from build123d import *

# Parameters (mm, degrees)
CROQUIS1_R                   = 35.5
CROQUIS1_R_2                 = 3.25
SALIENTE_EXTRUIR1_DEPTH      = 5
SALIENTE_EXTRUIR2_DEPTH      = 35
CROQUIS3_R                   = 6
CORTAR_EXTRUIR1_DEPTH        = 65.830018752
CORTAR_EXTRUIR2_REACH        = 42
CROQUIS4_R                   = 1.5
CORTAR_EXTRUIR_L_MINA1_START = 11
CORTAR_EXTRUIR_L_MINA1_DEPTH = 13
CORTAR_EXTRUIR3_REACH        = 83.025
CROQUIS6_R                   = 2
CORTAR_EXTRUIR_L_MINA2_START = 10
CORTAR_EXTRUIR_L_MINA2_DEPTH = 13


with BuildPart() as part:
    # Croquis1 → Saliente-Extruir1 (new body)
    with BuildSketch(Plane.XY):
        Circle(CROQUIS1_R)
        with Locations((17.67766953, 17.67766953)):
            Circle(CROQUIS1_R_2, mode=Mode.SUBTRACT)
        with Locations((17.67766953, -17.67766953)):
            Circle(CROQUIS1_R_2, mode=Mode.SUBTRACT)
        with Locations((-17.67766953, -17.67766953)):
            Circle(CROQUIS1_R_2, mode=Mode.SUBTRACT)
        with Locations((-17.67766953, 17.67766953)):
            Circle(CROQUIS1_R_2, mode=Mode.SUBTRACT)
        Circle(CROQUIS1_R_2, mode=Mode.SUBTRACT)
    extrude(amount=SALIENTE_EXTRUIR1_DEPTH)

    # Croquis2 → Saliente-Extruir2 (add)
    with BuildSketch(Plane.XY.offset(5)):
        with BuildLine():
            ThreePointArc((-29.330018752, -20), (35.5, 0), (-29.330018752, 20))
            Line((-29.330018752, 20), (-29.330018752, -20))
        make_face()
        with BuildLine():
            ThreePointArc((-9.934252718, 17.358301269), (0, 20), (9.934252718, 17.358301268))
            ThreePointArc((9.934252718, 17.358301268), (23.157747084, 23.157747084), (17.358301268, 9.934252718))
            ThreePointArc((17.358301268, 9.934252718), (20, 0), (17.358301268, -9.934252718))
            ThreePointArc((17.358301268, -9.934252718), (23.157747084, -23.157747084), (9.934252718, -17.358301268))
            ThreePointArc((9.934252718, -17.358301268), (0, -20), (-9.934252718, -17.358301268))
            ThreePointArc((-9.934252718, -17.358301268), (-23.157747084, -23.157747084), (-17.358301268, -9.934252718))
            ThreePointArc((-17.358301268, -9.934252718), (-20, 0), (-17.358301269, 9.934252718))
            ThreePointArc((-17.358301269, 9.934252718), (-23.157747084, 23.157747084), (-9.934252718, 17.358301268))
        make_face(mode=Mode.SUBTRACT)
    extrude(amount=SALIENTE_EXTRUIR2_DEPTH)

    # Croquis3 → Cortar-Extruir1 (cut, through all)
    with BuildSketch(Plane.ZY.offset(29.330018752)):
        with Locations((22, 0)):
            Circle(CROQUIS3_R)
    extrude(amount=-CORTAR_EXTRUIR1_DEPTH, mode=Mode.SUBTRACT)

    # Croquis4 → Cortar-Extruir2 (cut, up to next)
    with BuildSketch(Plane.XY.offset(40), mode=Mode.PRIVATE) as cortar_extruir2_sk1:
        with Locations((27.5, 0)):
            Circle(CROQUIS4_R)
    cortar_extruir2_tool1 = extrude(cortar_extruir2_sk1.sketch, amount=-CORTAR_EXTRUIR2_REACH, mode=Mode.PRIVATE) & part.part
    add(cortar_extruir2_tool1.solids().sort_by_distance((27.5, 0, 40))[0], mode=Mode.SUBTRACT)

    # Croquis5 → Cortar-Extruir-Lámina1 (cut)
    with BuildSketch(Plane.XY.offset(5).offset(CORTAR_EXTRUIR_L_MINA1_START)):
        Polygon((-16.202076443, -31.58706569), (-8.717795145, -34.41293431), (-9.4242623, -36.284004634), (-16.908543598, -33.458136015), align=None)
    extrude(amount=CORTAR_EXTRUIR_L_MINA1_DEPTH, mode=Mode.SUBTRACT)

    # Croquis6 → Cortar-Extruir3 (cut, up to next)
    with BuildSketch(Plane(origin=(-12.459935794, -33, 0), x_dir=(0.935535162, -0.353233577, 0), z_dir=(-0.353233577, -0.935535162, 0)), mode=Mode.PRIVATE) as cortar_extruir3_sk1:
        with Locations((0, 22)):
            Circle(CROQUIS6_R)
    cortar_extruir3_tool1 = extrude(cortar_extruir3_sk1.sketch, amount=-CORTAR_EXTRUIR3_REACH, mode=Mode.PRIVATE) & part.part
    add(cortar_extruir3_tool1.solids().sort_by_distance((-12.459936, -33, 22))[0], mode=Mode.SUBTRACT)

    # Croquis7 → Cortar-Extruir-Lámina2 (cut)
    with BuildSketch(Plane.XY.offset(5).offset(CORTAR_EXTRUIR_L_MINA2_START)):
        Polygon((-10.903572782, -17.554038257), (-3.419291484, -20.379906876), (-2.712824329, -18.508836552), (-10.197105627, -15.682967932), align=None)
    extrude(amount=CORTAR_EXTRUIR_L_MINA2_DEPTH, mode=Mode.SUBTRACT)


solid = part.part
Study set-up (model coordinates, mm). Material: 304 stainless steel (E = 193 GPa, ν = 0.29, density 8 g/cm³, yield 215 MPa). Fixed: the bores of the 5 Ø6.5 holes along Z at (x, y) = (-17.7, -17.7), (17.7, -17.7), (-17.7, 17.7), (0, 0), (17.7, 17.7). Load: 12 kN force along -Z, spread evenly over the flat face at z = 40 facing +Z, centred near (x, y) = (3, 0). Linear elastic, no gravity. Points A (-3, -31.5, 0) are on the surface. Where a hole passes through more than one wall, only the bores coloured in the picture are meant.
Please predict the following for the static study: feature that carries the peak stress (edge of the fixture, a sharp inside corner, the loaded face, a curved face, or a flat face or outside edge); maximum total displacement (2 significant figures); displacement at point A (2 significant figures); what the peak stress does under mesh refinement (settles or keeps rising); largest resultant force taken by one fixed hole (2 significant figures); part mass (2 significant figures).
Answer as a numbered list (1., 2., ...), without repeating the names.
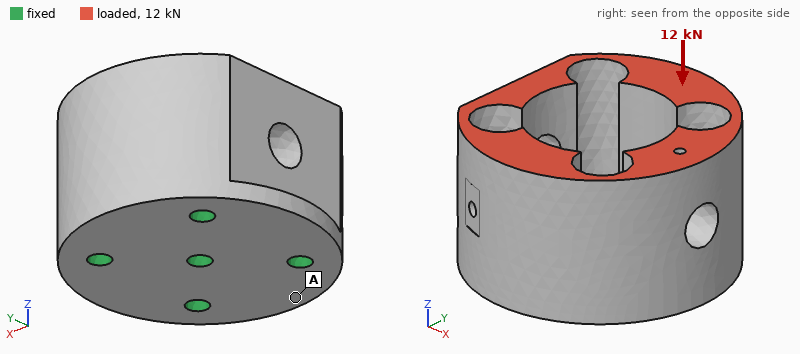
1. edge of the fixture
2. 6.2 µm
3. 4.4 µm
4. keeps rising
5. 3.3 kN
6. 650 g
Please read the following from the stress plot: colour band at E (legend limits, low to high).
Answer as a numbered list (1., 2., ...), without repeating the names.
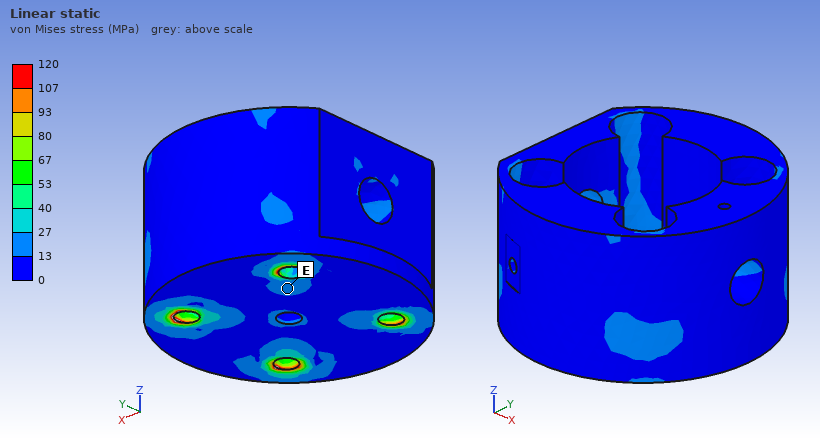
1. 13 to 27 MPa
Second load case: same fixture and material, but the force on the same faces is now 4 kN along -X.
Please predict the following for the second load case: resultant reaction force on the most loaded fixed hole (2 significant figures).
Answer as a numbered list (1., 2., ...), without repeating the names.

1. 2.2 kN
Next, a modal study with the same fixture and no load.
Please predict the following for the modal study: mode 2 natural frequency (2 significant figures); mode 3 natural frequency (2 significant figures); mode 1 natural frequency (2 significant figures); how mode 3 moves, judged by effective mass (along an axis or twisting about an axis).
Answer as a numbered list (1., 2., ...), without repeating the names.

1. 5500 Hz
2. 5900 Hz
3. 5400 Hz
4. along X
